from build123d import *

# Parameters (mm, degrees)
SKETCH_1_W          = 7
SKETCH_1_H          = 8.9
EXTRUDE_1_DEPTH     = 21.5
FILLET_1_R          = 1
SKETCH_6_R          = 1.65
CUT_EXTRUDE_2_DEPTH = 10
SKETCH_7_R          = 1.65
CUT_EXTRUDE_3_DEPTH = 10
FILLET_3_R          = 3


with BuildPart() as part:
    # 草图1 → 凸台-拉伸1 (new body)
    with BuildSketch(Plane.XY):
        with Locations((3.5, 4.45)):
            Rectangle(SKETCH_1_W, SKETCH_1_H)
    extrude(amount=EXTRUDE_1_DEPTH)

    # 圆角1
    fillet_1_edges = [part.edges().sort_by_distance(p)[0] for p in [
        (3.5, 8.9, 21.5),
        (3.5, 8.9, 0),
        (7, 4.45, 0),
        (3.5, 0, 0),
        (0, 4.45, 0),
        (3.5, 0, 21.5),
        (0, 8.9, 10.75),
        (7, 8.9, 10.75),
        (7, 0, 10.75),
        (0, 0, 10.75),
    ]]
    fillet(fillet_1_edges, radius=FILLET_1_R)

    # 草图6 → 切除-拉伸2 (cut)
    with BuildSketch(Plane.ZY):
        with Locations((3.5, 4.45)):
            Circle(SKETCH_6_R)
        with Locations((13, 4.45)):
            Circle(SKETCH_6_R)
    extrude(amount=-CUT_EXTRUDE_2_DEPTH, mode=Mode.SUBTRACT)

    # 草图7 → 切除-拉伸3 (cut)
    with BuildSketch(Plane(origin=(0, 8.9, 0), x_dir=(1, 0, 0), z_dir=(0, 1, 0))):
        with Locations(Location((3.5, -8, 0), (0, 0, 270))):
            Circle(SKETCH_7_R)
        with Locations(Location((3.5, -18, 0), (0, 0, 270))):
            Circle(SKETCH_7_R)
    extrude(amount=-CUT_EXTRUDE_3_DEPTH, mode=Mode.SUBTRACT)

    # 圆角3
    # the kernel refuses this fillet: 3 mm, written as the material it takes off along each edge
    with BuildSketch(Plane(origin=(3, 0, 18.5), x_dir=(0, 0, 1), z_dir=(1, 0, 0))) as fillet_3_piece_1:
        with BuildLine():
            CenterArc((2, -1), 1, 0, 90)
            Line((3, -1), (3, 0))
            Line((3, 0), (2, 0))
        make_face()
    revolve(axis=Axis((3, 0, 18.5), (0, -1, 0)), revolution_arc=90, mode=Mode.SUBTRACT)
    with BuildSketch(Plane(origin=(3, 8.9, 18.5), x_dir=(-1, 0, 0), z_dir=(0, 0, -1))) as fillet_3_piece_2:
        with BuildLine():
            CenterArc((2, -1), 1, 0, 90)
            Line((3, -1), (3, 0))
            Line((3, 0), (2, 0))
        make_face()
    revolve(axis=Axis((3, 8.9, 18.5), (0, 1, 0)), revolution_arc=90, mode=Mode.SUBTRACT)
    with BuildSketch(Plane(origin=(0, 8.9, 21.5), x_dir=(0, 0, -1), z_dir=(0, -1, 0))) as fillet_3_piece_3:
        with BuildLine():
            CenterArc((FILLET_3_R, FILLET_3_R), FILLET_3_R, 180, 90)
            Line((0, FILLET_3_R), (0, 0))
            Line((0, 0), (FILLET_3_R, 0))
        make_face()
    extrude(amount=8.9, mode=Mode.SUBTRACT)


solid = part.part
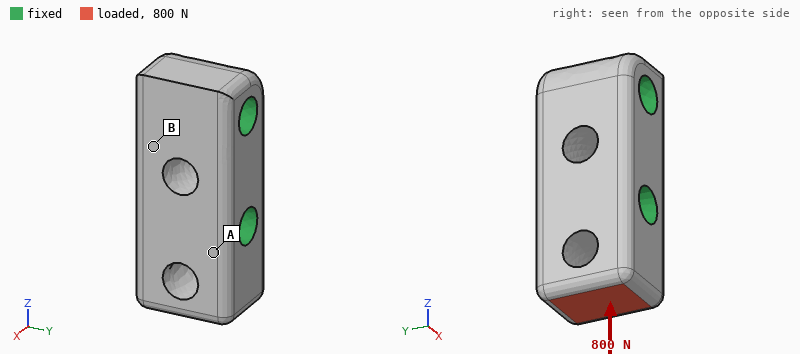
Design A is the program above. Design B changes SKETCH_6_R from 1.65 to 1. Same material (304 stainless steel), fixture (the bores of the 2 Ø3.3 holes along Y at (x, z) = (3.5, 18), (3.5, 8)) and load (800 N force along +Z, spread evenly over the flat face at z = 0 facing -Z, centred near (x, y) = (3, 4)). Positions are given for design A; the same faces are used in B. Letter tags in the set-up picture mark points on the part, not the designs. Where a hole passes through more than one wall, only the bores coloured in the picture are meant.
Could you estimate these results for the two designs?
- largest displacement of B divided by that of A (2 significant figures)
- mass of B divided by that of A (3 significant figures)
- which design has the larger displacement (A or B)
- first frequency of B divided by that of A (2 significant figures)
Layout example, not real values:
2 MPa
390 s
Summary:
0.65
1.07
A
1.0
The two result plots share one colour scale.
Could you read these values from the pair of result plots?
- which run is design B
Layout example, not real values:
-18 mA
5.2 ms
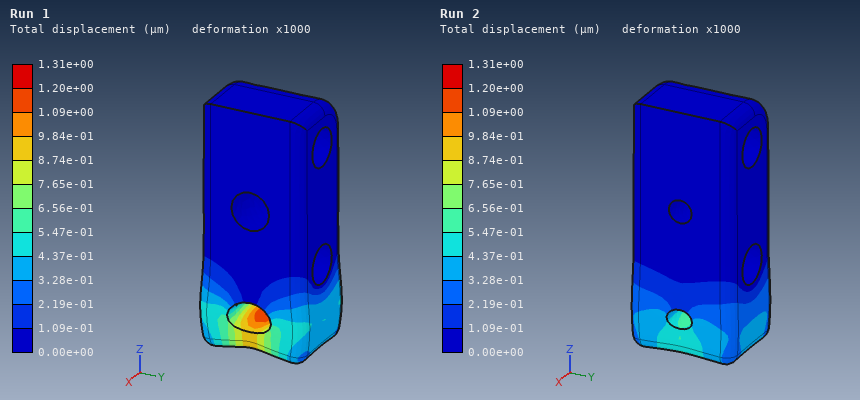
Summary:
Run 2
